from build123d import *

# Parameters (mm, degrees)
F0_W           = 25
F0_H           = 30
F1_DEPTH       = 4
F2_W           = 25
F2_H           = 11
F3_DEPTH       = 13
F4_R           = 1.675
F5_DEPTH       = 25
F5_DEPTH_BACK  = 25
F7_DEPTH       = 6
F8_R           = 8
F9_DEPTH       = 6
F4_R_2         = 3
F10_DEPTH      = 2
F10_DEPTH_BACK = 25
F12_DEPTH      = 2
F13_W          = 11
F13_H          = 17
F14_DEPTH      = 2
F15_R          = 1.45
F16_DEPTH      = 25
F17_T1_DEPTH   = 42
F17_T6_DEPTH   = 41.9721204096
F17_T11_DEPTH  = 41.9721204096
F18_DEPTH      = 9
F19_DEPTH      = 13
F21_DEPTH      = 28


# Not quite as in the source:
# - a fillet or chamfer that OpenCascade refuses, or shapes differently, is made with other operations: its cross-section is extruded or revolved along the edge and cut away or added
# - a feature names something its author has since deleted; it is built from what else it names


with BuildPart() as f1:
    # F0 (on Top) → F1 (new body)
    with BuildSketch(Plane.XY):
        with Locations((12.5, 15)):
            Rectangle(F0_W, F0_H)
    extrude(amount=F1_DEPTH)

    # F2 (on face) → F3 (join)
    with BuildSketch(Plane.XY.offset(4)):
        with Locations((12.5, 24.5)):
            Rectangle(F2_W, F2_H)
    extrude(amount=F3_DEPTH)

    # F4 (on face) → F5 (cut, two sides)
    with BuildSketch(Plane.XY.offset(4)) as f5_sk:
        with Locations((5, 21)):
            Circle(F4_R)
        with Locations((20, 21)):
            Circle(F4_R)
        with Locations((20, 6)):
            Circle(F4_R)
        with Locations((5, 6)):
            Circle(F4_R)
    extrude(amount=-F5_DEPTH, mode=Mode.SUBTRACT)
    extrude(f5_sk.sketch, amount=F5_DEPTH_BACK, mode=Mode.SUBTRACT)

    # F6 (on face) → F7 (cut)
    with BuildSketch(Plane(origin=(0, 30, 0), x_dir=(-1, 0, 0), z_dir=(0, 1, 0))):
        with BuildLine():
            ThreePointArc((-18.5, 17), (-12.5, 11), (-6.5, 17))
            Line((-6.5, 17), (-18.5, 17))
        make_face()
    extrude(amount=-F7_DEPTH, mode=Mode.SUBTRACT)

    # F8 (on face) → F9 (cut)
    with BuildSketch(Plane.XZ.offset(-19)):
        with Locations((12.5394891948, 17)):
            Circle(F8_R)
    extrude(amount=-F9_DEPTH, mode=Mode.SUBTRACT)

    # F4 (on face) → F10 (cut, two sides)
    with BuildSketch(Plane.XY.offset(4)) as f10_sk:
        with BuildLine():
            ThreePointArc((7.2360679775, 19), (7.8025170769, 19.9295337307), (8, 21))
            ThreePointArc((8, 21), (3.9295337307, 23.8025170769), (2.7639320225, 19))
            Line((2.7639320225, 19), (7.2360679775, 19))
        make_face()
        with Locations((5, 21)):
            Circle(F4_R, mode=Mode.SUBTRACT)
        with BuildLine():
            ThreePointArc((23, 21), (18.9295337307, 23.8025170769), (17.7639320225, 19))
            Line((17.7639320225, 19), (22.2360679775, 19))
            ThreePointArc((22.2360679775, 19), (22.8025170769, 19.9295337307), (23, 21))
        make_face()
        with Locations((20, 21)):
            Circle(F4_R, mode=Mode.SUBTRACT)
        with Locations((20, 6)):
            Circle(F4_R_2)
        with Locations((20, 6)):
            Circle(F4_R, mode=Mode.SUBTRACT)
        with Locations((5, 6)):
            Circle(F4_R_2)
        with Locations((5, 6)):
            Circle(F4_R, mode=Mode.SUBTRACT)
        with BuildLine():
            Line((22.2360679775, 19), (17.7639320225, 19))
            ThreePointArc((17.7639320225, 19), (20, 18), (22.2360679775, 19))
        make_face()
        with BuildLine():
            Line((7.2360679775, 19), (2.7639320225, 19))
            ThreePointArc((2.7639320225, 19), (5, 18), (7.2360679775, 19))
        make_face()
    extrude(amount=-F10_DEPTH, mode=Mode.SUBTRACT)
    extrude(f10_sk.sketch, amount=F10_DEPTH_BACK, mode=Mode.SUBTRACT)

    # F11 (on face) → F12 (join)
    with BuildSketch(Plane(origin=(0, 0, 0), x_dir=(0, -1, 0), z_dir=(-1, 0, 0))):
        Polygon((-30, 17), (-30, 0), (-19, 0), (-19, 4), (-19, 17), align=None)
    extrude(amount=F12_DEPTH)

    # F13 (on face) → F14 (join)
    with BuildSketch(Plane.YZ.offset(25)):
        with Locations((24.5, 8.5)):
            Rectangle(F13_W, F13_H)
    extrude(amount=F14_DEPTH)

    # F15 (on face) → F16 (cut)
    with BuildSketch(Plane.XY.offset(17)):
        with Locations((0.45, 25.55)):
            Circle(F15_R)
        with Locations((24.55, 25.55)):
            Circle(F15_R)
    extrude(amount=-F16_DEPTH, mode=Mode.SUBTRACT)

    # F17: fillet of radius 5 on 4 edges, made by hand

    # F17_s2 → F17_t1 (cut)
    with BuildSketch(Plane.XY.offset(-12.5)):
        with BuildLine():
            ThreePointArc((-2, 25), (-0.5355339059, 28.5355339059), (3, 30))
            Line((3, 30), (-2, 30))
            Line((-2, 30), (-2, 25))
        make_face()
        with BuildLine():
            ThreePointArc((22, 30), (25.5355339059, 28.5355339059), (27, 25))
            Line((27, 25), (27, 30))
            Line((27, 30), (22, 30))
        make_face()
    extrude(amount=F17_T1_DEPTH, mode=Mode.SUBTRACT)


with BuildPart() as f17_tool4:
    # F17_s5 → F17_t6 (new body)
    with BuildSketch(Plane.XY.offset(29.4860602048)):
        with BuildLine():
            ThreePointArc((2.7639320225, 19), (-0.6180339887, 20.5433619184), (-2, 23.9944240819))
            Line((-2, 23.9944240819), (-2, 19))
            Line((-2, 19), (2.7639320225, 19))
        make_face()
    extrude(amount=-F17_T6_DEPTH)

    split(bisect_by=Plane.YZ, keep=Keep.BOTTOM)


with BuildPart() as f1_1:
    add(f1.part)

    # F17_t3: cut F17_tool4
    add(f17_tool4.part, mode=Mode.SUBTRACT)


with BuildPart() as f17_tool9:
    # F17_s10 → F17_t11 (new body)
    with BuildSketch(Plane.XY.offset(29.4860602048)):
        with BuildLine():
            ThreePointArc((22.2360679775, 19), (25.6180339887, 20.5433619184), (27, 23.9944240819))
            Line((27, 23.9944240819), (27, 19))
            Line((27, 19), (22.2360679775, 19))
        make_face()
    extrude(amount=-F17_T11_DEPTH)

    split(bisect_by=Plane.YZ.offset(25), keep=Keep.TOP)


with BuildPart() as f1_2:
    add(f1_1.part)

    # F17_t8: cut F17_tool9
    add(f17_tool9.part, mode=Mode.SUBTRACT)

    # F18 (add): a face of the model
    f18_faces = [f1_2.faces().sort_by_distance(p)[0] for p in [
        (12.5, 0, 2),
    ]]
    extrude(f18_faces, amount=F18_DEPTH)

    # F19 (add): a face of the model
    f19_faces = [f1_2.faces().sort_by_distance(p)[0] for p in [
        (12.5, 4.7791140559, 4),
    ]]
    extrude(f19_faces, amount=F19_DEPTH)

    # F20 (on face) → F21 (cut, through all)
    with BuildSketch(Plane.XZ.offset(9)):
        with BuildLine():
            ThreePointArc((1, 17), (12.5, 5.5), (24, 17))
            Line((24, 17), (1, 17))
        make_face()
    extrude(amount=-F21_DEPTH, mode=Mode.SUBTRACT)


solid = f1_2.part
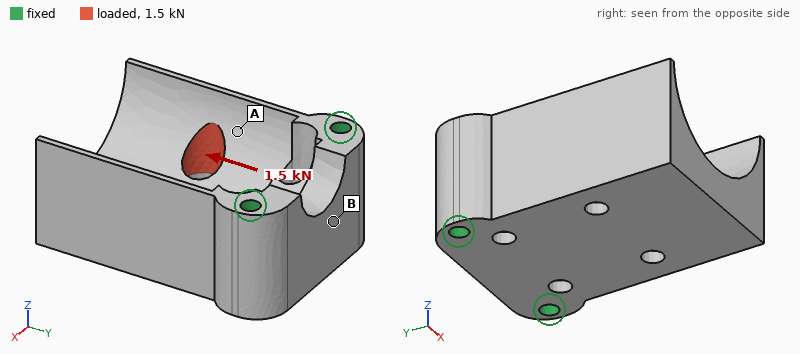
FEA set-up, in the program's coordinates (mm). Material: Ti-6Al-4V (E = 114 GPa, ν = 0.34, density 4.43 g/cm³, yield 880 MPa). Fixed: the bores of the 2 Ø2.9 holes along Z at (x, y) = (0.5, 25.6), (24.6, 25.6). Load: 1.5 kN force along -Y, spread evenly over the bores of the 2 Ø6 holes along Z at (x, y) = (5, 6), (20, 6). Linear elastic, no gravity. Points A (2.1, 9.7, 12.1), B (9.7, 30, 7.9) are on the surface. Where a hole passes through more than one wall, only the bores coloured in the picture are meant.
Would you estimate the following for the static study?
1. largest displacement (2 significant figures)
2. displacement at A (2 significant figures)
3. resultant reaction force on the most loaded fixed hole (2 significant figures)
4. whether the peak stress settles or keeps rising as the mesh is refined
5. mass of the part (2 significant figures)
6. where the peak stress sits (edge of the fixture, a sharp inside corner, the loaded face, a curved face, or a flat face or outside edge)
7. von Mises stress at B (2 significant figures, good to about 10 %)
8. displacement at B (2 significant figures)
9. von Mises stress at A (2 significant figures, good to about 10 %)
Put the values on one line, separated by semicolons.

3.1 µm; 1.7 µm; 760 N; keeps rising; 40 g; edge of the fixture; 4.1 MPa; 0.60 µm; 15 MPa
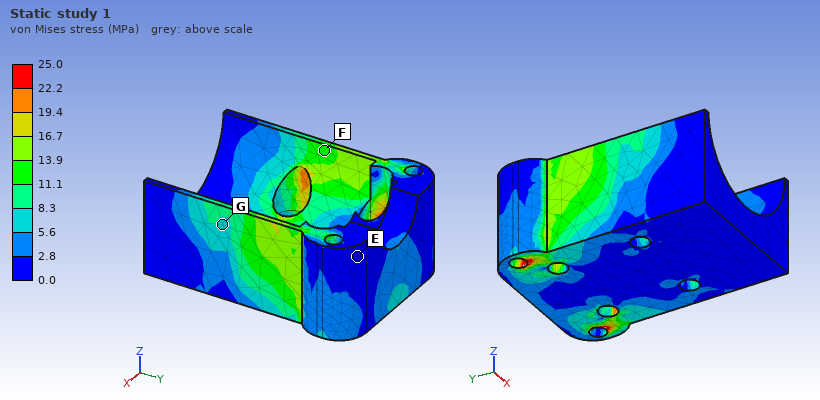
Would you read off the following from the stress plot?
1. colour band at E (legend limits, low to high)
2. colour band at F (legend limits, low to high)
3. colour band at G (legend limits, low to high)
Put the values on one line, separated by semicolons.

0.0 to 2.8 MPa; 11.1 to 13.9 MPa; 5.6 to 8.3 MPa
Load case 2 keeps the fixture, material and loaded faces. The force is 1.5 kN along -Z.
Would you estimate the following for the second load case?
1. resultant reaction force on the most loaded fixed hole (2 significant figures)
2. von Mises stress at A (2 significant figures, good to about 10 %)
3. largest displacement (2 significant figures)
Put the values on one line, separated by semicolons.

750 N; 29 MPa; 30 µm
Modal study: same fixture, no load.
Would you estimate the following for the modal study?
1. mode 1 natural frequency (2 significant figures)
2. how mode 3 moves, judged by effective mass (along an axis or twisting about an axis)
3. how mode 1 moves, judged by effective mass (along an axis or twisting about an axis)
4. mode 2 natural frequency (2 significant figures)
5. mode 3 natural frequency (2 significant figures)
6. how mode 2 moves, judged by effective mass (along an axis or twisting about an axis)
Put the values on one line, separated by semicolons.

7800 Hz; along X; along Z; 9700 Hz; 16 kHz; along X
